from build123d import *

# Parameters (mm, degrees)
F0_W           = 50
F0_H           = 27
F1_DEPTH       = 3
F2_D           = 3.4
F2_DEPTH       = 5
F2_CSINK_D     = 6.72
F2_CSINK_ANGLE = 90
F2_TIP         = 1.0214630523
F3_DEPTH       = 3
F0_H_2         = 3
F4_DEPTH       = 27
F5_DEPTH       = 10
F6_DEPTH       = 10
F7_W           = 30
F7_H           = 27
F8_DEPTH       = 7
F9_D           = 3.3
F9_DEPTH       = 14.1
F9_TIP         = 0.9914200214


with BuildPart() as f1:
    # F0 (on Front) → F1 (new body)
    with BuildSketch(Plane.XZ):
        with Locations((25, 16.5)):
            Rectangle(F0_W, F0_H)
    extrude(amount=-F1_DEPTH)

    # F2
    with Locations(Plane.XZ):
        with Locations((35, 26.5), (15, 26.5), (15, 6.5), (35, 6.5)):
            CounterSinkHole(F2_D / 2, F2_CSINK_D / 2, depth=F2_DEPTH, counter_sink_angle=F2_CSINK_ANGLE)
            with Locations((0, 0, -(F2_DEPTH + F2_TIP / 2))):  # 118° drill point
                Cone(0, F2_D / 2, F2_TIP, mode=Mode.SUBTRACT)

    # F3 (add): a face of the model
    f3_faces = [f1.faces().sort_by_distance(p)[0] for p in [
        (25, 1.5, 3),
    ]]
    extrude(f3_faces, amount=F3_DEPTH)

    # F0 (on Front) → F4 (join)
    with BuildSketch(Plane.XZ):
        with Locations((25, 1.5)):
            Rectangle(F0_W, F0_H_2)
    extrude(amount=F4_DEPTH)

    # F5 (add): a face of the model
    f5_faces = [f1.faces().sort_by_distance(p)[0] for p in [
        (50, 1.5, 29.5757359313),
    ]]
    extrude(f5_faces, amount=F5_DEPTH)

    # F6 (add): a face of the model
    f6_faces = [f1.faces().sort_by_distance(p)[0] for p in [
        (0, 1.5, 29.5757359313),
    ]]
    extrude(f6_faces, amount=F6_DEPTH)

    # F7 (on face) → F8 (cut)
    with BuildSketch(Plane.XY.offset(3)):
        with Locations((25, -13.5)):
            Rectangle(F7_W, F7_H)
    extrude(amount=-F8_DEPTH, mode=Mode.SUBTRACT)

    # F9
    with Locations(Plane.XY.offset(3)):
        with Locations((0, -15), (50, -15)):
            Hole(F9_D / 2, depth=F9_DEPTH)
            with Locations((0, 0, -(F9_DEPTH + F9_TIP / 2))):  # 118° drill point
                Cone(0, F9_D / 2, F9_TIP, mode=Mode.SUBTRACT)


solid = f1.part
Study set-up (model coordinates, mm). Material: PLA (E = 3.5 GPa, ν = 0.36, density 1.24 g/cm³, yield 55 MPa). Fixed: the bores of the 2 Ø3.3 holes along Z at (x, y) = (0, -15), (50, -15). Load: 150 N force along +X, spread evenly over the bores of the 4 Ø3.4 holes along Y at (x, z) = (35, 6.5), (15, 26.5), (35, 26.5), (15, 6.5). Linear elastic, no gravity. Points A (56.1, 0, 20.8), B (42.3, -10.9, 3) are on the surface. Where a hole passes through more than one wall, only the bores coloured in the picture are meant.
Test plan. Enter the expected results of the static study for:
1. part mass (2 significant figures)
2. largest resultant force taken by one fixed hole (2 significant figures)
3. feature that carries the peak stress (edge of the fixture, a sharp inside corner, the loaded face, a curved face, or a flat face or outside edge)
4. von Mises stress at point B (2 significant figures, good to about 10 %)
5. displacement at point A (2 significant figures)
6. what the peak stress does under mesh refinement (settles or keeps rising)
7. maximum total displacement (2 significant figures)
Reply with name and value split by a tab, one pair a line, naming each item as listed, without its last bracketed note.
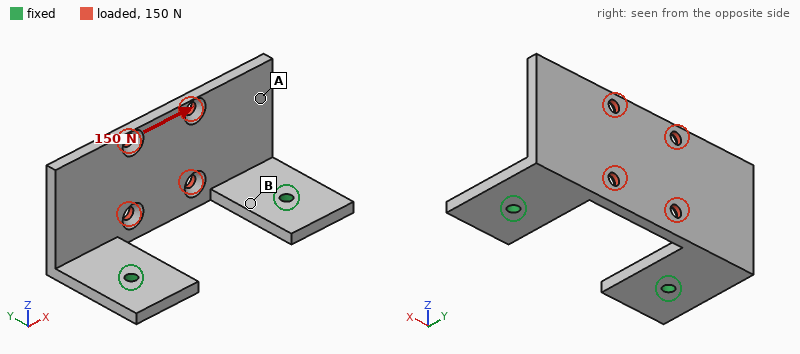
part mass	12 g
largest resultant force taken by one fixed hole	87 N
feature that carries the peak stress	edge of the fixture
von Mises stress at point B	8.0 MPa
displacement at point A	0.46 mm
what the peak stress does under mesh refinement	keeps rising
maximum total displacement	0.59 mm
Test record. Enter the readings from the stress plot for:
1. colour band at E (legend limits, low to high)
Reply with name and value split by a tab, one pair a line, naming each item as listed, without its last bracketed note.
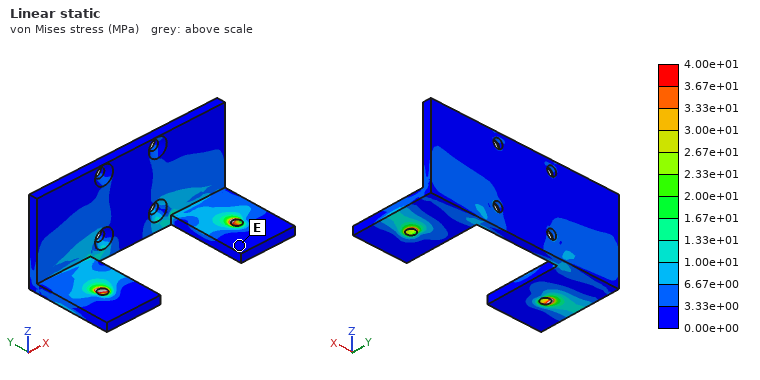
colour band at E	0.00e+00 to 3.33e+00 MPa
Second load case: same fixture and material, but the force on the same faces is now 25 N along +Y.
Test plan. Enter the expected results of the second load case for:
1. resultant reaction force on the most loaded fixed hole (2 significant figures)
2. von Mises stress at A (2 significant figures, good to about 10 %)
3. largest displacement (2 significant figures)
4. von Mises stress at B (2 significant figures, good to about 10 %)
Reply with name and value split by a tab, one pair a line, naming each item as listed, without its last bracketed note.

resultant reaction force on the most loaded fixed hole	14 N
von Mises stress at A	1.3 MPa
largest displacement	0.84 mm
von Mises stress at B	5.5 MPa
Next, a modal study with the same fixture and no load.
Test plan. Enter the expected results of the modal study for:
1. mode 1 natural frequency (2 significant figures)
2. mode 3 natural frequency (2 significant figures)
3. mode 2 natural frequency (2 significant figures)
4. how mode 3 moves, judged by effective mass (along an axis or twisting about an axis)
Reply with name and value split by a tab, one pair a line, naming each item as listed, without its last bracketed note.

mode 1 natural frequency	410 Hz
mode 3 natural frequency	1300 Hz
mode 2 natural frequency	800 Hz
how mode 3 moves, judged by effective mass	along Z
